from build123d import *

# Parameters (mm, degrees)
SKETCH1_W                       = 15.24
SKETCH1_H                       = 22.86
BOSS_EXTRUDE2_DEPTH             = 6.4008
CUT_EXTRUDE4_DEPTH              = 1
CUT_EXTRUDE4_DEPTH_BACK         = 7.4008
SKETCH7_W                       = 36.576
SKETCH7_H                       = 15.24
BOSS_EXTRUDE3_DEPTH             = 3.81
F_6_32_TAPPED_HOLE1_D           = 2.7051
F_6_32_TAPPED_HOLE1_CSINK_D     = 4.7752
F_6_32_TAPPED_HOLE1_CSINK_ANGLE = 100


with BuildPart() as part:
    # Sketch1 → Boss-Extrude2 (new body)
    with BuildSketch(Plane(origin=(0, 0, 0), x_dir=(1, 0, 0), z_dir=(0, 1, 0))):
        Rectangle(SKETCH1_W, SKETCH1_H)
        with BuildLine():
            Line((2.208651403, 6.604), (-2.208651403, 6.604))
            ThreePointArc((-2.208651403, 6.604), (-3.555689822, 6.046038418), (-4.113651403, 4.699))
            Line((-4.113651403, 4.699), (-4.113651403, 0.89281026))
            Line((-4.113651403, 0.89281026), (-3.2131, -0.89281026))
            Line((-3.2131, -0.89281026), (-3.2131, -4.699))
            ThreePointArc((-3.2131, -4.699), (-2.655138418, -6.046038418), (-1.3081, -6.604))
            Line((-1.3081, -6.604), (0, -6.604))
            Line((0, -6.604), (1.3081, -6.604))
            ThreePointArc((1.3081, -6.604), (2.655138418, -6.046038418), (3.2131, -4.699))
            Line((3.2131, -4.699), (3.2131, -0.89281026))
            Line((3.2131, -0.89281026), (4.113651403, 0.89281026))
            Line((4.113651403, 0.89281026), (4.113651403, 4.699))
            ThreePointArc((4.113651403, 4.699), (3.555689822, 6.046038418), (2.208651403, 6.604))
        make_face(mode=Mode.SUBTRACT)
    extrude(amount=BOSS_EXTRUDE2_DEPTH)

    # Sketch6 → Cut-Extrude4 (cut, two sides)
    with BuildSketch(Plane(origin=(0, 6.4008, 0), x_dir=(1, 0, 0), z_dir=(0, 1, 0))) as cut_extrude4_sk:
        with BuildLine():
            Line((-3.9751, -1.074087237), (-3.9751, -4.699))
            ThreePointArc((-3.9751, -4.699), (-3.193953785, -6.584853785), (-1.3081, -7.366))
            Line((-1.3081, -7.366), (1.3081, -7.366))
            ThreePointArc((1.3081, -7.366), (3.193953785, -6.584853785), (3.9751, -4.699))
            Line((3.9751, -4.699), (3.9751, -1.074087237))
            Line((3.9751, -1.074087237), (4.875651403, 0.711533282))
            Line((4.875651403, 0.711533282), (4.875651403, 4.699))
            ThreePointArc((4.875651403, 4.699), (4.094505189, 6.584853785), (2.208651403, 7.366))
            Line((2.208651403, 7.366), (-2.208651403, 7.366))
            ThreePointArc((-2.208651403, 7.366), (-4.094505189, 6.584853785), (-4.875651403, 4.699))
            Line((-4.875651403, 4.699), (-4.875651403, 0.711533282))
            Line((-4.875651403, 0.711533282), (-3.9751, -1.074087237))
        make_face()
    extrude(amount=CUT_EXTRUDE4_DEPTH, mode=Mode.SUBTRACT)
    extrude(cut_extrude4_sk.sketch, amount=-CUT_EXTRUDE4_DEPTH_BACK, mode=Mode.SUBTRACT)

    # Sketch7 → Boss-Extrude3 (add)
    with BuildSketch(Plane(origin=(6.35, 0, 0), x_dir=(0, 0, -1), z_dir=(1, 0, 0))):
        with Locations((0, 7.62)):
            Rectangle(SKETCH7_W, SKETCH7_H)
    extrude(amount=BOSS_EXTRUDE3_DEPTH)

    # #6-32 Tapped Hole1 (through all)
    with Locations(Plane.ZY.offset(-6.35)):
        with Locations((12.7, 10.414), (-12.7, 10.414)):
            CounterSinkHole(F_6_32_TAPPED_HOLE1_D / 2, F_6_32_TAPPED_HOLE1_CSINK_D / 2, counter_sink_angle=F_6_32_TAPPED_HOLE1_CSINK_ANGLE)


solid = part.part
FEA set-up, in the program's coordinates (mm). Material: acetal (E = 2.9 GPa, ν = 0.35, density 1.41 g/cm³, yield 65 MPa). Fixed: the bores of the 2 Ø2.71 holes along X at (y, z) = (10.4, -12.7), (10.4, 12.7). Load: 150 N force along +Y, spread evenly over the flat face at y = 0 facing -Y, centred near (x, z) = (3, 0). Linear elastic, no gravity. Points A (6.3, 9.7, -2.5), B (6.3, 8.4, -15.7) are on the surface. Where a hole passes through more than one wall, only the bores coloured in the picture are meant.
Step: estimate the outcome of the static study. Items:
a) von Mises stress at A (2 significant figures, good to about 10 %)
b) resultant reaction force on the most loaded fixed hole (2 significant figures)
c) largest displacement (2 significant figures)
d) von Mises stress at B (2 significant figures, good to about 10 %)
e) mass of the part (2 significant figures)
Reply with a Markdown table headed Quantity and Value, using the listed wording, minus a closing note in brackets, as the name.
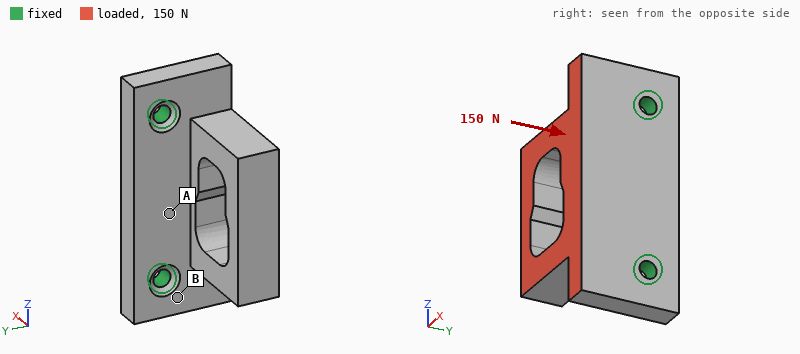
| Quantity | Value |
|---|---|
| von Mises stress at A | 4.1 MPa |
| resultant reaction force on the most loaded fixed hole | 79 N |
| largest displacement | 0.41 mm |
| von Mises stress at B | 9.2 MPa |
| mass of the part | 4.7 g |
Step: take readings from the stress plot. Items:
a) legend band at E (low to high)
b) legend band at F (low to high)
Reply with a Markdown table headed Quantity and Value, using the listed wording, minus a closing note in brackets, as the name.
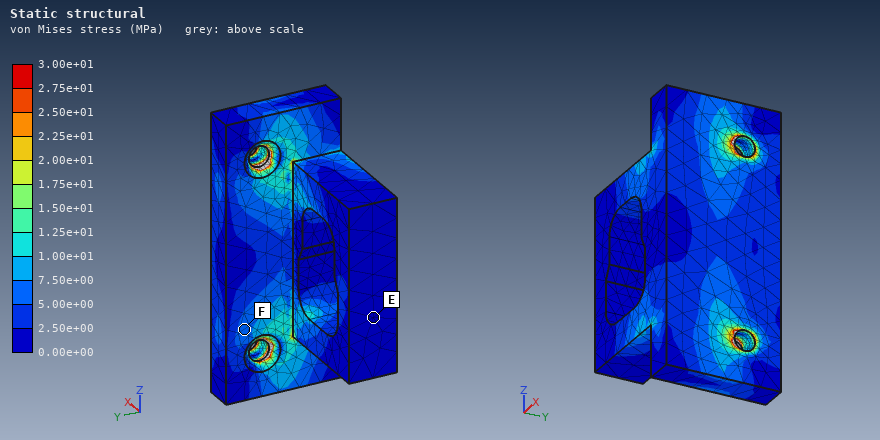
| Quantity | Value |
|---|---|
| legend band at E | 0.00e+00 to 2.50e+00 MPa |
| legend band at F | 5.00e+00 to 7.50e+00 MPa |
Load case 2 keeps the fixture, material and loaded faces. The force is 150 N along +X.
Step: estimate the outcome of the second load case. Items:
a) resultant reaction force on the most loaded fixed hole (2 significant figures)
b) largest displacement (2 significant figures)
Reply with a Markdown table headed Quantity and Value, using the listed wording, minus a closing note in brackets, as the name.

| Quantity | Value |
|---|---|
| resultant reaction force on the most loaded fixed hole | 76 N |
| largest displacement | 0.51 mm |
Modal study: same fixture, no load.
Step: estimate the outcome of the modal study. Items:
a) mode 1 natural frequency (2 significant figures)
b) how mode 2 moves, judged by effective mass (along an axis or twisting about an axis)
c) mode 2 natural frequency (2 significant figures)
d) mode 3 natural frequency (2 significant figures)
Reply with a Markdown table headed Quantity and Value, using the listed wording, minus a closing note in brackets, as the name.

| Quantity | Value |
|---|---|
| mode 1 natural frequency | 1900 Hz |
| how mode 2 moves, judged by effective mass | along Z |
| mode 2 natural frequency | 3900 Hz |
| mode 3 natural frequency | 5300 Hz |
